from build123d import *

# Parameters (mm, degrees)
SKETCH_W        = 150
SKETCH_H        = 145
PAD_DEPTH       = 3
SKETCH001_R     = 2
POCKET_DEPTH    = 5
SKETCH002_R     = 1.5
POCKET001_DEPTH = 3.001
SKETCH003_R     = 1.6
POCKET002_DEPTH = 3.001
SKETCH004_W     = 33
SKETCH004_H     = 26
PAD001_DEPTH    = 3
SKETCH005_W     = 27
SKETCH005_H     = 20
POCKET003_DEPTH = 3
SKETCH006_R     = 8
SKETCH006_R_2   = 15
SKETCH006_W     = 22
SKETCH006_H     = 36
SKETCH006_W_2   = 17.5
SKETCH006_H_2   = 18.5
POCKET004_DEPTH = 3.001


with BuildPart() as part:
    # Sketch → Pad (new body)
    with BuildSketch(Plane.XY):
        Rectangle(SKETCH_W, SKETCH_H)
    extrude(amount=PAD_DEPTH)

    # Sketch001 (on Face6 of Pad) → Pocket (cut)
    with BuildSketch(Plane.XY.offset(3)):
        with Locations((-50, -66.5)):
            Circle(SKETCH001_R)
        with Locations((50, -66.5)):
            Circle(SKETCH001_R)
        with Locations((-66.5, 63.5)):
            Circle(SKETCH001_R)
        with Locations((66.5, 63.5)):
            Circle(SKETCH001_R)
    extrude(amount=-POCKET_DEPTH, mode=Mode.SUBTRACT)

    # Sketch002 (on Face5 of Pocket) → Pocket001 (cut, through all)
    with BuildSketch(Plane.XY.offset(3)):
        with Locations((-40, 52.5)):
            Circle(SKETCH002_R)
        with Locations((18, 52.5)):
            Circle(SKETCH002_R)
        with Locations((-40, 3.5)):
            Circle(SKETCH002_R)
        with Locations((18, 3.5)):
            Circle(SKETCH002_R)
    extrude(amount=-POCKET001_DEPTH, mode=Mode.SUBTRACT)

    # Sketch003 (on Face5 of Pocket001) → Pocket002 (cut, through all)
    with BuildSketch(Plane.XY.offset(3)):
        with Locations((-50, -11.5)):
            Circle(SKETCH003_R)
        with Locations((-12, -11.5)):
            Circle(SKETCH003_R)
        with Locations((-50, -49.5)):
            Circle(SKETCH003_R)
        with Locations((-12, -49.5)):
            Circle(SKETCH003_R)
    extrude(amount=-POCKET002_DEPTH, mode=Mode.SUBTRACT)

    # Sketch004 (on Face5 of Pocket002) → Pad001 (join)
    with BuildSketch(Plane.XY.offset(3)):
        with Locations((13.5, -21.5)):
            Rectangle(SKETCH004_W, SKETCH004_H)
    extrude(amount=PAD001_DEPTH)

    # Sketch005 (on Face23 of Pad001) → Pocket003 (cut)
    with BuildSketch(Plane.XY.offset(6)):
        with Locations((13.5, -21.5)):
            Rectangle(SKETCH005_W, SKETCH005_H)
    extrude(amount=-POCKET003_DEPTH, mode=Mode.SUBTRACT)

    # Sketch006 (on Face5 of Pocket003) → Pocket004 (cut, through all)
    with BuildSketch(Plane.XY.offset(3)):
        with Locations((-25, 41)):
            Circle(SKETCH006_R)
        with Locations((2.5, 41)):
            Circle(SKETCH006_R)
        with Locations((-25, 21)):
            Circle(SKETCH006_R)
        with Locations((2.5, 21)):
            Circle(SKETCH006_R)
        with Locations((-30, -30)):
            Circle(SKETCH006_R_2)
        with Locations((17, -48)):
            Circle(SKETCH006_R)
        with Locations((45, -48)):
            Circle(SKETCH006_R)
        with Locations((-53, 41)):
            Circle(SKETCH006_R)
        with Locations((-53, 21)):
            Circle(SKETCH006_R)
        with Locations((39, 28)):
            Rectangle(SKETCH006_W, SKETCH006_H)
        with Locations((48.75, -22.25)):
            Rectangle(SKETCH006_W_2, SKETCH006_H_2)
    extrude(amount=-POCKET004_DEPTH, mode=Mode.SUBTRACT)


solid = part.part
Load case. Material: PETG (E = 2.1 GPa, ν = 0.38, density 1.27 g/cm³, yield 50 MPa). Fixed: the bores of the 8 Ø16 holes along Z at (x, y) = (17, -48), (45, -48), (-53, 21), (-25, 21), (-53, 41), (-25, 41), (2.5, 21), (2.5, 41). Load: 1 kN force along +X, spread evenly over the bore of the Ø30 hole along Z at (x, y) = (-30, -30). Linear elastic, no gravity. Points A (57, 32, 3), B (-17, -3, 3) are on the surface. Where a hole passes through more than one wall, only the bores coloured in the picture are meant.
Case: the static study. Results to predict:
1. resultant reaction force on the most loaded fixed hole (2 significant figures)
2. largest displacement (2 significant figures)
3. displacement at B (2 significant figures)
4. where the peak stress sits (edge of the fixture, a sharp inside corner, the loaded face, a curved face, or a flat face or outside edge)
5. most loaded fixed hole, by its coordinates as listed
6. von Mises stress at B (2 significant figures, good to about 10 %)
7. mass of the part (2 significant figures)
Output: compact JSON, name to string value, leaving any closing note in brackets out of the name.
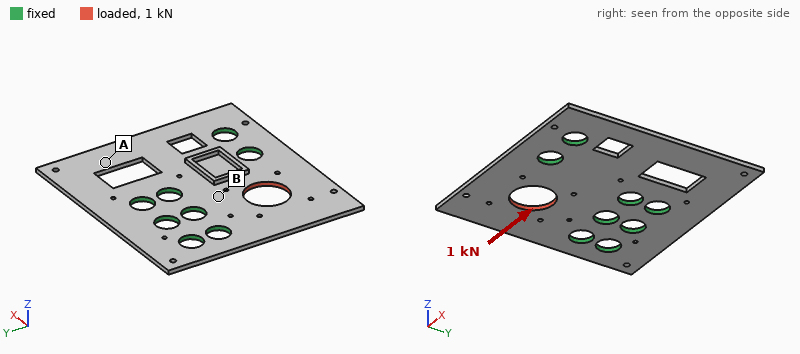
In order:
{"resultant reaction force on the most loaded fixed hole": "500 N", "largest displacement": "0.16 mm", "displacement at B": "0.039 mm", "where the peak stress sits": "a curved face", "most loaded fixed hole, by its coordinates as listed": "(17, -48)", "von Mises stress at B": "3.0 MPa", "mass of the part": "71 g"}
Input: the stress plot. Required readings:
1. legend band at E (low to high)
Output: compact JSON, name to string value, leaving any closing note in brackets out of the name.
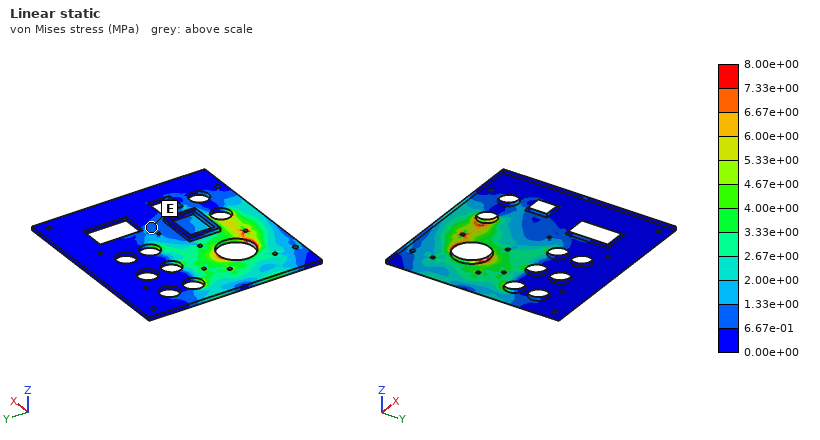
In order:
{"legend band at E": "6.67e-01 to 1.33e+00 MPa"}
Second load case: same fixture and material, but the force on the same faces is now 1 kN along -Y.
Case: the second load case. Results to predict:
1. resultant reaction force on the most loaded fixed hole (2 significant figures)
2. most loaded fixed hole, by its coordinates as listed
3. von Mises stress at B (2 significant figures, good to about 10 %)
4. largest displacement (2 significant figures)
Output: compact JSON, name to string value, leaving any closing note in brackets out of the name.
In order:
{"resultant reaction force on the most loaded fixed hole": "350 N", "most loaded fixed hole, by its coordinates as listed": "(-53, 21)", "von Mises stress at B": "3.4 MPa", "largest displacement": "0.16 mm"}
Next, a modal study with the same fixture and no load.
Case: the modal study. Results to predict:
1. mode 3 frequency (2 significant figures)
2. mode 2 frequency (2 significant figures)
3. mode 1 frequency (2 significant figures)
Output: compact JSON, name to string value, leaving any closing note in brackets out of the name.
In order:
{"mode 3 frequency": "360 Hz", "mode 2 frequency": "160 Hz", "mode 1 frequency": "160 Hz"}
